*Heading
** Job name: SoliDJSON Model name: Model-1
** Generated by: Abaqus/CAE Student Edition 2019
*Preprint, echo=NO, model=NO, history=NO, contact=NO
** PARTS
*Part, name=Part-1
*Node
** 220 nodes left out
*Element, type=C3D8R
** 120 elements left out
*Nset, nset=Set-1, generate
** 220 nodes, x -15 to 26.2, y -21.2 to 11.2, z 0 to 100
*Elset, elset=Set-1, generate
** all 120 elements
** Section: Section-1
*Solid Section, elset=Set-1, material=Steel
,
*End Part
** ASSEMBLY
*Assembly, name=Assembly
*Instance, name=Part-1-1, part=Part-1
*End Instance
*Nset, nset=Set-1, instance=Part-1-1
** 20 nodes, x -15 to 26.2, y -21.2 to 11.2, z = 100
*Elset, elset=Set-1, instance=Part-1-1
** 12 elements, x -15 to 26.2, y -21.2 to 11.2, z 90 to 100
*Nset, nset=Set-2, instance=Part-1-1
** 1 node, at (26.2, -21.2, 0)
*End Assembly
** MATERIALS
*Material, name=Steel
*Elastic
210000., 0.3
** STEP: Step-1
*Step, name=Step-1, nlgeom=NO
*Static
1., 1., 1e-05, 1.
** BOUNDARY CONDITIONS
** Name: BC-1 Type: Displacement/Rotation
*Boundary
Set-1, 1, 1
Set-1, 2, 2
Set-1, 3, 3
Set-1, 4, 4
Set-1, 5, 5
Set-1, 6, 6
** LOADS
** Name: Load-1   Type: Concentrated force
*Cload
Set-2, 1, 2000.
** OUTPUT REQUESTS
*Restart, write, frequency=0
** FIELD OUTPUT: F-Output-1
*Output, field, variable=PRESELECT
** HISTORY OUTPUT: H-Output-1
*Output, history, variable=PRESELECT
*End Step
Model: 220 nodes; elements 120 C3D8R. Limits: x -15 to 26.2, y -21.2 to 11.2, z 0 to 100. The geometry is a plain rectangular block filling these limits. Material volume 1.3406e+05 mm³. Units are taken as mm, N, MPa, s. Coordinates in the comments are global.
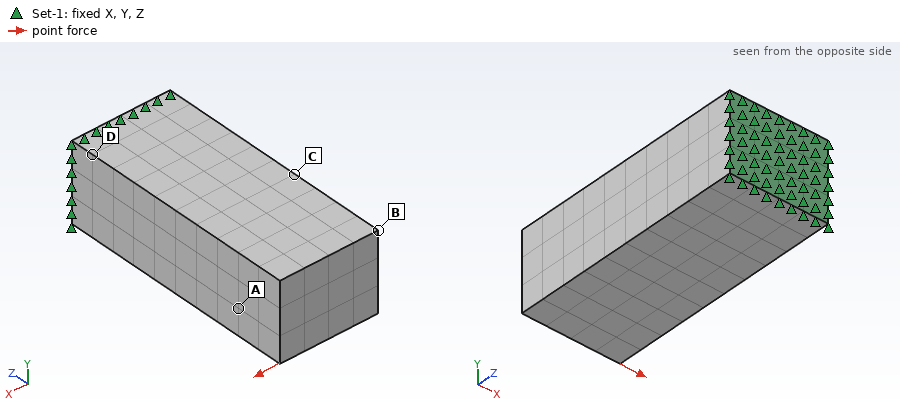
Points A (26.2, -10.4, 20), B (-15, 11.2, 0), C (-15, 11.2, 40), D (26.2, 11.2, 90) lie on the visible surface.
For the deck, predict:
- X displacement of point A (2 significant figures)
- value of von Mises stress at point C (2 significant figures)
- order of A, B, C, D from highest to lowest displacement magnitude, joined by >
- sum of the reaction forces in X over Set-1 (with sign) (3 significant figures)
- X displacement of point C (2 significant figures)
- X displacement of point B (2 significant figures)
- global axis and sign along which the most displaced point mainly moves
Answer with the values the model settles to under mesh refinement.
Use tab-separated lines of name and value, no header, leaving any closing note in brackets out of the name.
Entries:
X displacement of point A	0.014 mm
value of von Mises stress at point C	8.4 MPa
order of A, B, C, D from highest to lowest displacement magnitude, joined by >	B > A > C > D
sum of the reaction forces in X over Set-1 (with sign)	-2000 N
X displacement of point C	0.0068 mm
X displacement of point B	0.016 mm
global axis and sign along which the most displaced point mainly moves	+X
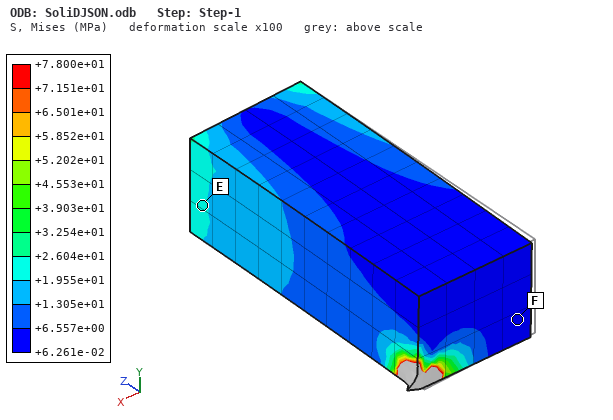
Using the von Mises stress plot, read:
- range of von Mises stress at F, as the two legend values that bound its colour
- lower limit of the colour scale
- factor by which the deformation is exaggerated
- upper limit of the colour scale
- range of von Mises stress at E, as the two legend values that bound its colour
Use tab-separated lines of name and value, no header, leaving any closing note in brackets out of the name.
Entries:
range of von Mises stress at F, as the two legend values that bound its colour	+6.261e-02 to +6.557e+00 MPa
lower limit of the colour scale	+6.261e-02 MPa
factor by which the deformation is exaggerated	100
upper limit of the colour scale	+7.800e+01 MPa
range of von Mises stress at E, as the two legend values that bound its colour	+1.955e+01 to +2.604e+01 MPa
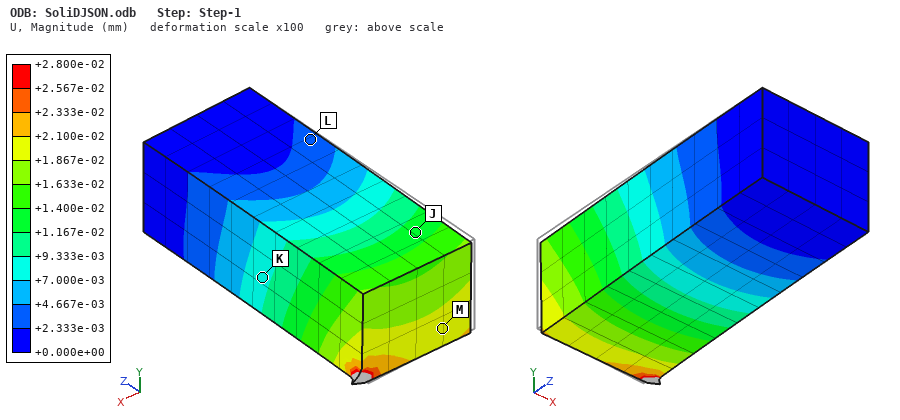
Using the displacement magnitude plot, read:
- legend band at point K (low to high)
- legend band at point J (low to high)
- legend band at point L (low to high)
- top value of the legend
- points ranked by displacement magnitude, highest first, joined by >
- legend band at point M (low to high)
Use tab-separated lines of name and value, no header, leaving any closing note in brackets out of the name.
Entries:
legend band at point K	+7.000e-03 to +9.333e-03 mm
legend band at point J	+1.167e-02 to +1.400e-02 mm
legend band at point L	+2.333e-03 to +4.667e-03 mm
top value of the legend	+2.800e-02 mm
points ranked by displacement magnitude, highest first, joined by >	M > J > K > L
legend band at point M	+1.867e-02 to +2.100e-02 mm
